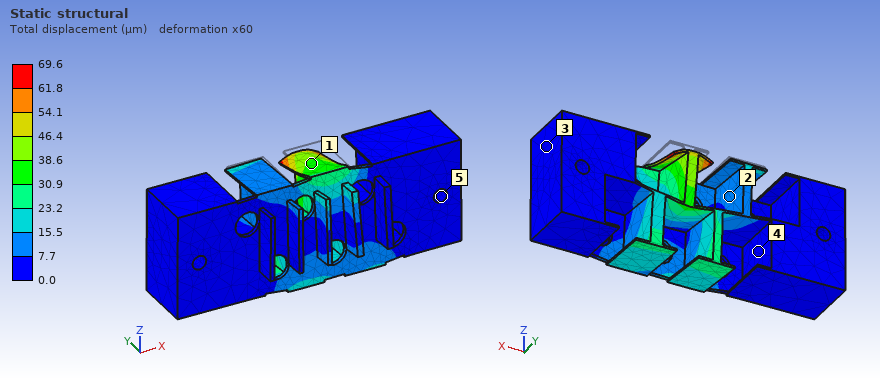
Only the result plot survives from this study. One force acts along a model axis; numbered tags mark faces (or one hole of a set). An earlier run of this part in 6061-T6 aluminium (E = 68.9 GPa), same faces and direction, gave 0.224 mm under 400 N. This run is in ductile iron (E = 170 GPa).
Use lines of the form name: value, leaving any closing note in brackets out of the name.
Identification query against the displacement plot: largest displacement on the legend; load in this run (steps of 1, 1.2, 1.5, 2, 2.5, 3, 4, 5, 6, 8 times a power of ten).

largest displacement on the legend: 69.6 µm
load in this run: 300 N
